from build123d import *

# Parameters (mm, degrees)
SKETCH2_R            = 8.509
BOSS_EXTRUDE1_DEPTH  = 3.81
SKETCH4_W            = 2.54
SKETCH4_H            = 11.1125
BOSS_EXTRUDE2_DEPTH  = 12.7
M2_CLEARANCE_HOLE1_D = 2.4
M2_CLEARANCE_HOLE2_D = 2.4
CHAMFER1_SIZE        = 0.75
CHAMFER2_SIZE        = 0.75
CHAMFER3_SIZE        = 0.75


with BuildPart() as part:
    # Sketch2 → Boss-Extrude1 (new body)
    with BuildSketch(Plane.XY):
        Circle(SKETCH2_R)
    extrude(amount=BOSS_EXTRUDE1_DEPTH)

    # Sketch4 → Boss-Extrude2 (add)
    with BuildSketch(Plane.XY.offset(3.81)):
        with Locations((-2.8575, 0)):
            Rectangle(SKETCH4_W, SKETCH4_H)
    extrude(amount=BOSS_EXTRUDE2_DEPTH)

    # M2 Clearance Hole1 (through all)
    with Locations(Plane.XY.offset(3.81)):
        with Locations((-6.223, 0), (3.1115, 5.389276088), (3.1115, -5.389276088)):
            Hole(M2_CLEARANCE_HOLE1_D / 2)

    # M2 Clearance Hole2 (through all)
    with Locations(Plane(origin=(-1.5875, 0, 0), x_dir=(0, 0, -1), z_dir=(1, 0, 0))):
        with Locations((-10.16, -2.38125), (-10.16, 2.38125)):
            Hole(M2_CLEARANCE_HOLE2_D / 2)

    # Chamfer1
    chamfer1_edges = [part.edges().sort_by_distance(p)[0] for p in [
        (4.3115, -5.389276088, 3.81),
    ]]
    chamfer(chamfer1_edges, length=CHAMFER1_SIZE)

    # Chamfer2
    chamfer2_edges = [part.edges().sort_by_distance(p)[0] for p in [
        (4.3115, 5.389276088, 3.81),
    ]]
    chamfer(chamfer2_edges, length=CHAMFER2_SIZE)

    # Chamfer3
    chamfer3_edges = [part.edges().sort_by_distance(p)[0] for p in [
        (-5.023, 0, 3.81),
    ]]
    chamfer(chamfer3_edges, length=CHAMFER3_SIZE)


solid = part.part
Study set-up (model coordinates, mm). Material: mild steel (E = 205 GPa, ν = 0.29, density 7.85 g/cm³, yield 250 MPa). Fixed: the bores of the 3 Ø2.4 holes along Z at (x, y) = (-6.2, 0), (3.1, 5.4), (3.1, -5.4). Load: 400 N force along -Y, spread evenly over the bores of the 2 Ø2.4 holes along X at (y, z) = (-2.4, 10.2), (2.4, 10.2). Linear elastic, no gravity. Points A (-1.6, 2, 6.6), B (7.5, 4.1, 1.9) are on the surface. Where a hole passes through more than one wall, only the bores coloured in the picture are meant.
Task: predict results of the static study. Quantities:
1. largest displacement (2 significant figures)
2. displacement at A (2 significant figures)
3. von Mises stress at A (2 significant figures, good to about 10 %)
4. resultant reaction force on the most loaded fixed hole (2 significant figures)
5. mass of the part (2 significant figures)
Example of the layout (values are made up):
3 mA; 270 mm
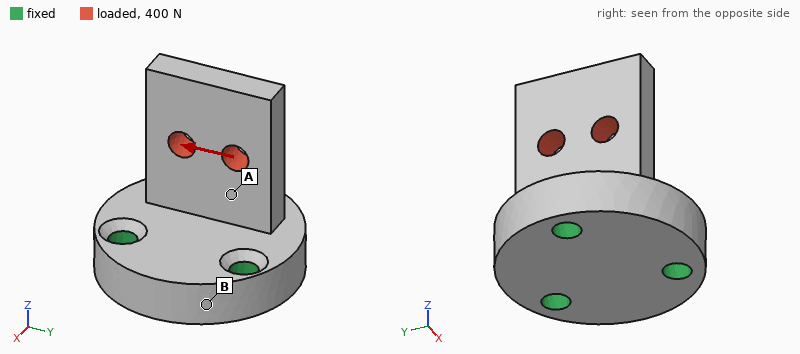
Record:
7.7 µm; 2.3 µm; 38 MPa; 230 N; 9.0 g
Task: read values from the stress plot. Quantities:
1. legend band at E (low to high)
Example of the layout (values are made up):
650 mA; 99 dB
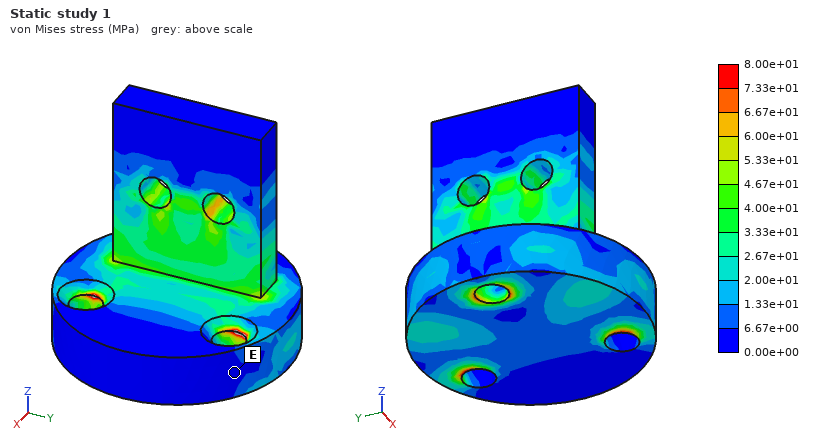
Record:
0.00e+00 to 6.67e+00 MPa
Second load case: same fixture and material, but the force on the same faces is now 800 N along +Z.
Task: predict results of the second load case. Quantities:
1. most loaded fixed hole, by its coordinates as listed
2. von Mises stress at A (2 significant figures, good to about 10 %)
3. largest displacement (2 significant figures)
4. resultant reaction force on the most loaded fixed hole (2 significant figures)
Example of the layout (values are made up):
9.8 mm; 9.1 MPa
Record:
(-6.2, 0); 29 MPa; 2.1 µm; 490 N
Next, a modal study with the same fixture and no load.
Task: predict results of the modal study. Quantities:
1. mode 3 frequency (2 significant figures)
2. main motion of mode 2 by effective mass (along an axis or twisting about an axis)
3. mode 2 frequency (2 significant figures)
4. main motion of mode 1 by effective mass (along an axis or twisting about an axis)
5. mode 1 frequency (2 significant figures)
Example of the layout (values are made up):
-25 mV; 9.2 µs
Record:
28 kHz; along Y; 25 kHz; along X; 11 kHz
